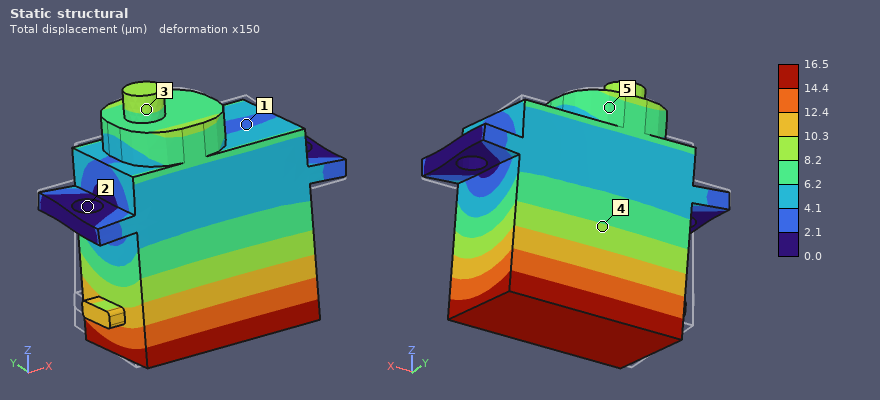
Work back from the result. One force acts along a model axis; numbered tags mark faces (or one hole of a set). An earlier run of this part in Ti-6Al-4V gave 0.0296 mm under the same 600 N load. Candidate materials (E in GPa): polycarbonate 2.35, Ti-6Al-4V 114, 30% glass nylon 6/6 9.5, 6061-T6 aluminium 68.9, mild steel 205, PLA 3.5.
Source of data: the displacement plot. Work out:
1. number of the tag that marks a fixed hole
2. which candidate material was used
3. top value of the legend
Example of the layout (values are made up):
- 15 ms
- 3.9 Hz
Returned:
- 2
- mild steel
- 16.5 µm
